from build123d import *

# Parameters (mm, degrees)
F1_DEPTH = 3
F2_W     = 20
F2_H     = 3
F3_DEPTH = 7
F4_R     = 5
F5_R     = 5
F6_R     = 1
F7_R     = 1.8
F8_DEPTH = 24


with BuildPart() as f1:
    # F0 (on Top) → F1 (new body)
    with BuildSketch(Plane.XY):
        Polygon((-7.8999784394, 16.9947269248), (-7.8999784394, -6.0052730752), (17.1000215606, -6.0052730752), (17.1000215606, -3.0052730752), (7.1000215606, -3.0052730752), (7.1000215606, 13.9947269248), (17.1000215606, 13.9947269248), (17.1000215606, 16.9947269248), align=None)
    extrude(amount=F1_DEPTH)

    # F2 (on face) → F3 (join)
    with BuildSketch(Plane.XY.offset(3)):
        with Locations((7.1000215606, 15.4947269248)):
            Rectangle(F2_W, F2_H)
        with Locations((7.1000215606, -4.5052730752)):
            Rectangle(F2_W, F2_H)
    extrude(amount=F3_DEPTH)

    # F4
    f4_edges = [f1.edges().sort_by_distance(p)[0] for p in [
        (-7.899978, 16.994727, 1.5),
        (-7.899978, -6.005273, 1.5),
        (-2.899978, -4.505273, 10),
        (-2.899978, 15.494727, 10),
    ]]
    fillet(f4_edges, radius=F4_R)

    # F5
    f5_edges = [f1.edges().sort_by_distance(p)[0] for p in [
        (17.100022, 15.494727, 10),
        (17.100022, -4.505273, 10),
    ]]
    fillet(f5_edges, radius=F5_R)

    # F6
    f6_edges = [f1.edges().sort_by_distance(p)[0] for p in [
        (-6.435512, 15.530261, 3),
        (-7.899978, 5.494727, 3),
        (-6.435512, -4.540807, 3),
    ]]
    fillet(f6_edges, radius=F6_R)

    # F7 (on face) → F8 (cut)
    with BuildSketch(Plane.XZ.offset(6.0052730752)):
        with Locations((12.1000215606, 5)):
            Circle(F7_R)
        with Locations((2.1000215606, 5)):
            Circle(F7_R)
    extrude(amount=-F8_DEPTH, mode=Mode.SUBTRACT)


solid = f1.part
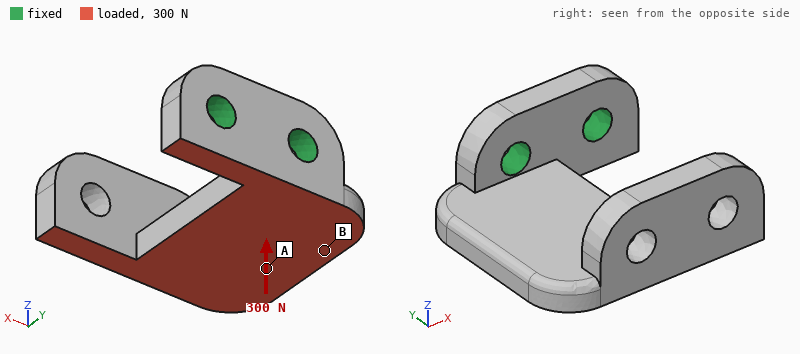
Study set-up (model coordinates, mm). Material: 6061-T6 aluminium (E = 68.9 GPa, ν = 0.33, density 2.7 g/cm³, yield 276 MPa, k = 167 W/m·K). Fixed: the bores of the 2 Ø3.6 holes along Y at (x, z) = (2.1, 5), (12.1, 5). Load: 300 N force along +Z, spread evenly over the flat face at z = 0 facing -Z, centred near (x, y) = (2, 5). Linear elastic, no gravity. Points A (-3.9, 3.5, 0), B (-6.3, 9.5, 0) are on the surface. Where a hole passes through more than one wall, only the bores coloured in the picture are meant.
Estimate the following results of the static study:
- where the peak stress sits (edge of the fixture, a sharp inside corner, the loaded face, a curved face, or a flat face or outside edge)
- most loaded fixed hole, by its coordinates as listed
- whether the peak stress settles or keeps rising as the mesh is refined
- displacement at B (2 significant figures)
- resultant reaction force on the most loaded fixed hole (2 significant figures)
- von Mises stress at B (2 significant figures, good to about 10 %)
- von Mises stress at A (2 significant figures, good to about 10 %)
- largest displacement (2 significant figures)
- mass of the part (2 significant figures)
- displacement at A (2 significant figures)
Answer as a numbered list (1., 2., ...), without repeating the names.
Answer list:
1. edge of the fixture
2. (2.1, 5)
3. keeps rising
4. 0.051 mm
5. 300 N
6. 54 MPa
7. 28 MPa
8. 0.26 mm
9. 4.9 g
10. 0.11 mm
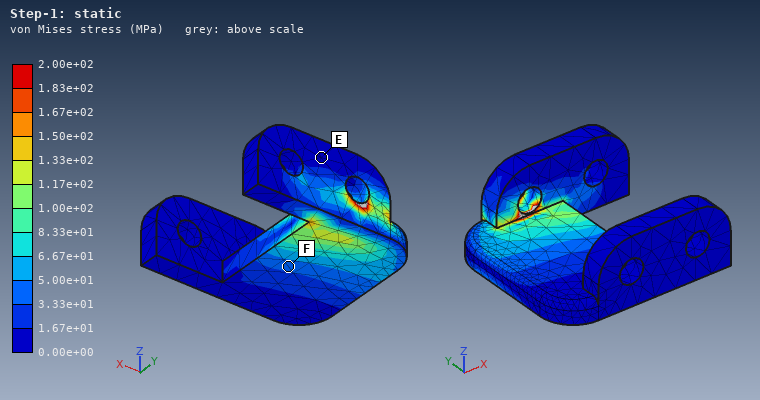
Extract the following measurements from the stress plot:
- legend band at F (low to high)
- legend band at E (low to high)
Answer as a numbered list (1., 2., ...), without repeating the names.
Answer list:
1. 3.33e+01 to 5.00e+01 MPa
2. 0.00e+00 to 1.67e+01 MPa
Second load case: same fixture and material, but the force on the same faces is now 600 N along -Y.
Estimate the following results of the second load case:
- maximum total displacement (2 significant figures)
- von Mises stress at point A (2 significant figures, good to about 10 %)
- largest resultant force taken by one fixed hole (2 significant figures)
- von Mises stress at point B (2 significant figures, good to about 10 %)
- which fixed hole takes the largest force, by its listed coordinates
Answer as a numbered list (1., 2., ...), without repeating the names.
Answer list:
1. 0.12 mm
2. 20 MPa
3. 560 N
4. 23 MPa
5. (2.1, 5)
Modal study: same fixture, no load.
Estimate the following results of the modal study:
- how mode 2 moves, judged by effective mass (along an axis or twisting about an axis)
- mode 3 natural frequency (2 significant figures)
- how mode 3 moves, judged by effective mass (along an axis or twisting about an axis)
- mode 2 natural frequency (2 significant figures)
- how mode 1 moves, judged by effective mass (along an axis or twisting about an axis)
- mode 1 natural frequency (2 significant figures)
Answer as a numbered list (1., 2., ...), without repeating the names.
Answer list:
1. along X
2. 7500 Hz
3. along X
4. 5000 Hz
5. along Z
6. 2700 Hz
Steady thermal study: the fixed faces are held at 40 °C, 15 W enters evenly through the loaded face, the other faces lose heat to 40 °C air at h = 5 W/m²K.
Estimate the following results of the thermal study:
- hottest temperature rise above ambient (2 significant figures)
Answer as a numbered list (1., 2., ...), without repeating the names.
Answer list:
1. 29 K
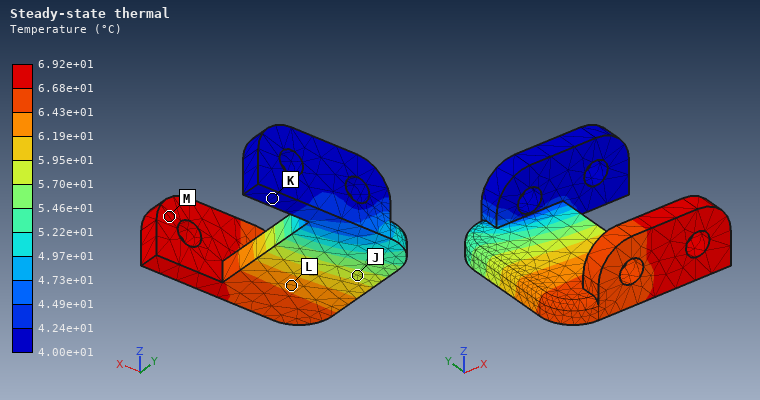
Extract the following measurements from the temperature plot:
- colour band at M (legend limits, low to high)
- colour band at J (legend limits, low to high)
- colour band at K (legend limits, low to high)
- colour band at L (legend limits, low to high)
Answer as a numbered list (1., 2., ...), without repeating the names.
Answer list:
1. 6.68e+01 to 6.92e+01 °C
2. 5.70e+01 to 5.95e+01 °C
3. 4.00e+01 to 4.24e+01 °C
4. 6.19e+01 to 6.43e+01 °C
